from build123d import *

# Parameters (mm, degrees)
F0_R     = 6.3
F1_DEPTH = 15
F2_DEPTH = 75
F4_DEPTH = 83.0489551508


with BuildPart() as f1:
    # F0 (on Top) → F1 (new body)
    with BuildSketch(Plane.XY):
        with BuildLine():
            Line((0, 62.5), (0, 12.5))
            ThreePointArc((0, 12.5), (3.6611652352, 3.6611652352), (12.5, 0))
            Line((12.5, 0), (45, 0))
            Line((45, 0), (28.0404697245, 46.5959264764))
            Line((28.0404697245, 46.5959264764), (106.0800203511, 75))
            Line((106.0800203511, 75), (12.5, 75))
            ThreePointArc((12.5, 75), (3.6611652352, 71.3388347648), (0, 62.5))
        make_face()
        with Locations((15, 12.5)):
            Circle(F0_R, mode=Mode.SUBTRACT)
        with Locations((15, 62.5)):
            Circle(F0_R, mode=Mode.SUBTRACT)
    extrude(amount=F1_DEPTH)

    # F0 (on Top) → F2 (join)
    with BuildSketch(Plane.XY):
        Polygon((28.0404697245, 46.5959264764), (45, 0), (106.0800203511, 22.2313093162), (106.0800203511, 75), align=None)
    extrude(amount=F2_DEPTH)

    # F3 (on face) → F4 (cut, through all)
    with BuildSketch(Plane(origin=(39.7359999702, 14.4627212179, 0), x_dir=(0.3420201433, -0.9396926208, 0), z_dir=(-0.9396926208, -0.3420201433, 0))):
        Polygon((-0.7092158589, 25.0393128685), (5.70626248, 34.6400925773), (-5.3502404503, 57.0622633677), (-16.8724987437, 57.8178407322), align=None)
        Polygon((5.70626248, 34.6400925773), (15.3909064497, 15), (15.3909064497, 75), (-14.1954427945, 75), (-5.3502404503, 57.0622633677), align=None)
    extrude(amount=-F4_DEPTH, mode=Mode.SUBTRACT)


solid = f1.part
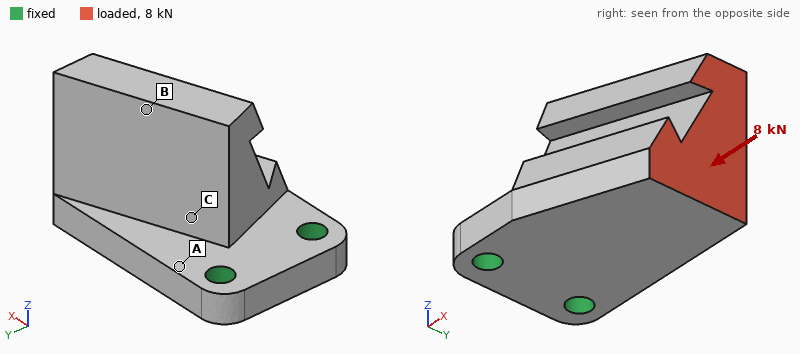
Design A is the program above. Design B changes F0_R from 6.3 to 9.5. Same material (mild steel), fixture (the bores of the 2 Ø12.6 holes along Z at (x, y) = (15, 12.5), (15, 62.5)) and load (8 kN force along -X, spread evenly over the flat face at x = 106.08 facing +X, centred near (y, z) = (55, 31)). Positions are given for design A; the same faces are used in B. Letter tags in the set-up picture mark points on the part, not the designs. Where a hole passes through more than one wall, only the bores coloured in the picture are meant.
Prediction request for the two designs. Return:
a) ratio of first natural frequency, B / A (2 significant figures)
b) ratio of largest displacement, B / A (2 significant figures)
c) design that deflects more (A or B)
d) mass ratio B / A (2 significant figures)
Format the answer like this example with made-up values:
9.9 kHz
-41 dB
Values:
1.1
0.84
A
0.98
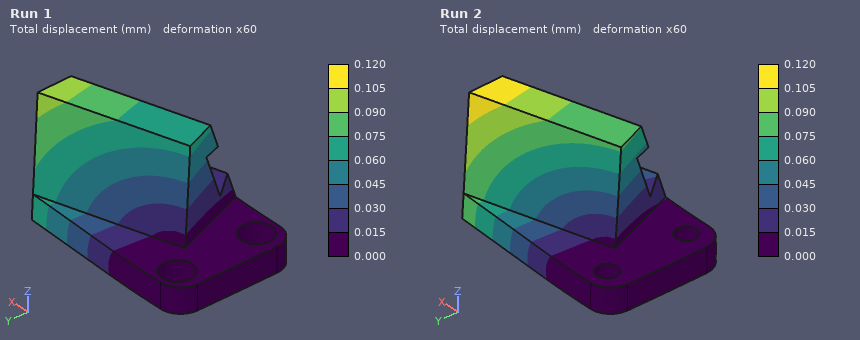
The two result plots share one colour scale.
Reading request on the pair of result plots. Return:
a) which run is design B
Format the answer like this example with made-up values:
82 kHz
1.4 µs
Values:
Run 1
